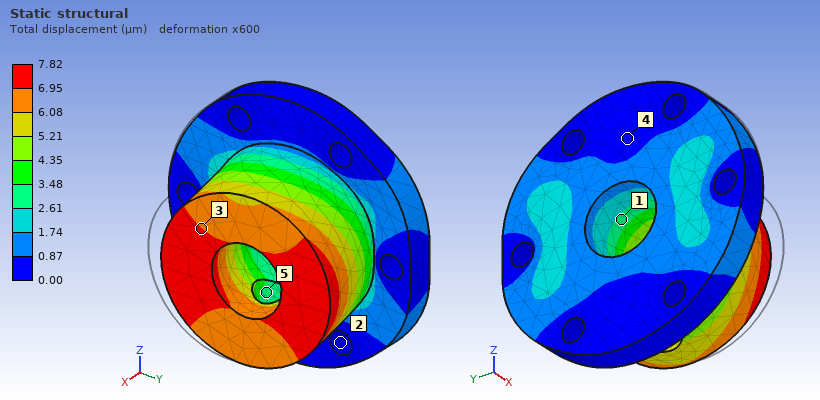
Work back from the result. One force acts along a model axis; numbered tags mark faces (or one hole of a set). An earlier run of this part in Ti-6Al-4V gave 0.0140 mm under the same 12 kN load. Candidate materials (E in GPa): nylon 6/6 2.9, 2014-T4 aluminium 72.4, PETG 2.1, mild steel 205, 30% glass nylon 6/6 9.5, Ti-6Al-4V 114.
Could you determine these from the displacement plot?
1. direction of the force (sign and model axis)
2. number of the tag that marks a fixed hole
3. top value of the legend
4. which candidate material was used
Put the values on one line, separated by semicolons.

+Y; 2; 7.82 µm; mild steel
